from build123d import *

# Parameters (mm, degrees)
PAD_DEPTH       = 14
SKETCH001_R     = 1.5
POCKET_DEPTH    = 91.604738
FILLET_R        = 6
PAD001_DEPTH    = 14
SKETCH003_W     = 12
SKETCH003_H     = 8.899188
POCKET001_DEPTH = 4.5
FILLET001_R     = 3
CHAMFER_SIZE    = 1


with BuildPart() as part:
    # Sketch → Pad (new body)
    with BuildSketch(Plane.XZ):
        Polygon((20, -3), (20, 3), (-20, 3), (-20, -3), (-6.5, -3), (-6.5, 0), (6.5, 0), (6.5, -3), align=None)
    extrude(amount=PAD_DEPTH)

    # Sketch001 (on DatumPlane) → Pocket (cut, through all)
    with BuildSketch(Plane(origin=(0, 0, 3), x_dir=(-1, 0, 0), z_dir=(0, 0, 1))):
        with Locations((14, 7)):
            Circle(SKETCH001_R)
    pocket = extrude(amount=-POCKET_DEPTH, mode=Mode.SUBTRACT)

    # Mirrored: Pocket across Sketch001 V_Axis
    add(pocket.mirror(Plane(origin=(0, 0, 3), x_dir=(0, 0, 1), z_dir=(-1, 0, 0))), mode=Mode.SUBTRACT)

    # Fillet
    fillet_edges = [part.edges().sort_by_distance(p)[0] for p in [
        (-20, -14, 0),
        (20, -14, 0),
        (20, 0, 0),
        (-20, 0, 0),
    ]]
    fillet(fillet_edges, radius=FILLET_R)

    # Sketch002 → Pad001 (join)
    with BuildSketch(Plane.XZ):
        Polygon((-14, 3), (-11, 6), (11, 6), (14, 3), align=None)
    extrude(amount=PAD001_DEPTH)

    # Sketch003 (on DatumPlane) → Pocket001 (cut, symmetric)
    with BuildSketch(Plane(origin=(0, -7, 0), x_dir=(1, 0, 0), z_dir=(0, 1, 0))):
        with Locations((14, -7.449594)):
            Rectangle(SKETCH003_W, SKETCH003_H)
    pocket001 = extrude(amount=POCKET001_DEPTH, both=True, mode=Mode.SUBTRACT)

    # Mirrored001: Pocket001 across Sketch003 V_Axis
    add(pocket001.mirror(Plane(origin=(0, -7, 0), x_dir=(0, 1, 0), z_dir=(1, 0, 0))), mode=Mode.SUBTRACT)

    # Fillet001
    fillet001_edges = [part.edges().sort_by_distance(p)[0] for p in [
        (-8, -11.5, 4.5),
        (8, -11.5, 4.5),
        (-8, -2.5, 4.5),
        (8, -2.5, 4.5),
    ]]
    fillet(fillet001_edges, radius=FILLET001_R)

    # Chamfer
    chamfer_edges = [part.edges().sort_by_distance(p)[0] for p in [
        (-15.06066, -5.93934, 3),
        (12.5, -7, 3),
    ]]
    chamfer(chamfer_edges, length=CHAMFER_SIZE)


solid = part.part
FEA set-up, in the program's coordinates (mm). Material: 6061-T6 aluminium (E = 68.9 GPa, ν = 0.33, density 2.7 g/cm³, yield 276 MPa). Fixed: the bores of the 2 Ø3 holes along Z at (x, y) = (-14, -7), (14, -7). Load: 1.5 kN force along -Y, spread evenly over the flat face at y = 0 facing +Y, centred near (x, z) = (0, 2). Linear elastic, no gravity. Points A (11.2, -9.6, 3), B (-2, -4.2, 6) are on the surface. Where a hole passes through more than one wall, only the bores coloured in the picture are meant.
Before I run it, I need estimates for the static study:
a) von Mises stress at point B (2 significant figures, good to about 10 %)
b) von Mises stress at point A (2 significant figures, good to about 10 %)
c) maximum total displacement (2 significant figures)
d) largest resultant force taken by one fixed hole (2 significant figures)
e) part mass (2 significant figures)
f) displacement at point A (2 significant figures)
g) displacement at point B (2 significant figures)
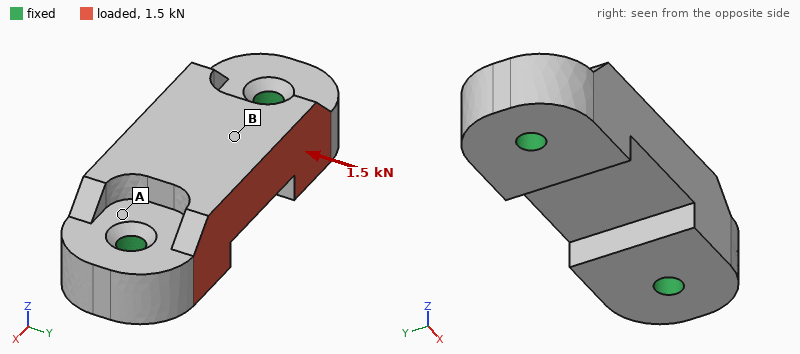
7.2 MPa
26 MPa
12 µm
750 N
9.1 g
3.3 µm
11 µm
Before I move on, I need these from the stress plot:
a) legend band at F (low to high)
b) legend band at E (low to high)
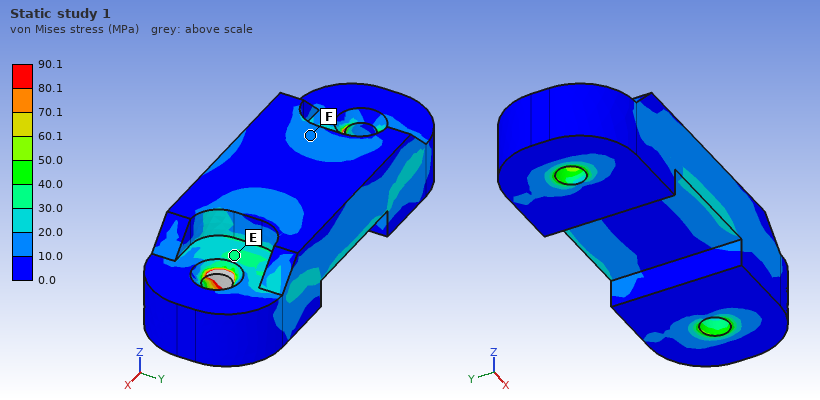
10.0 to 20.0 MPa
30.0 to 40.0 MPa
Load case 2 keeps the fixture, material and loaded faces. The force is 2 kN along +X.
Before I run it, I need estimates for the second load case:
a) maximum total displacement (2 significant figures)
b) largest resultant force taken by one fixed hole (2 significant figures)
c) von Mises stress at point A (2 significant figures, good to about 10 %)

6.5 µm
1.1 kN
8.5 MPa
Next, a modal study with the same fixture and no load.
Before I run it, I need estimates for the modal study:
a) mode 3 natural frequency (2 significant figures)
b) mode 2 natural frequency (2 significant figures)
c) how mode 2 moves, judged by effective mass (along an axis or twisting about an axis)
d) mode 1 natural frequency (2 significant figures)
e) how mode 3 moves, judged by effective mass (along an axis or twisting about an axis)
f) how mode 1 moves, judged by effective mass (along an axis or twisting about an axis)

41 kHz
30 kHz
along Z
24 kHz
along Y
along Y
